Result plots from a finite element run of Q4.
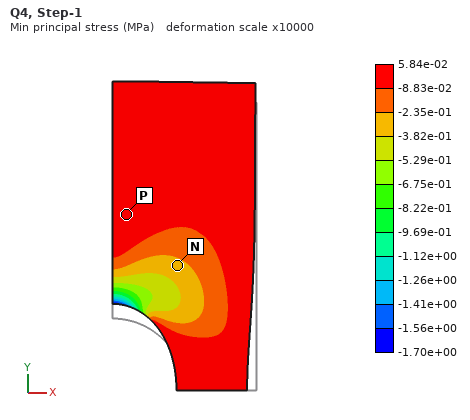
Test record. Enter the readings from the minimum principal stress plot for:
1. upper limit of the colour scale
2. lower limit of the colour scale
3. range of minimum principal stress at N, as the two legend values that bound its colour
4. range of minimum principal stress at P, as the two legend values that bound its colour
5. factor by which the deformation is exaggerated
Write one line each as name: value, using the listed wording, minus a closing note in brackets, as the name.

upper limit of the colour scale: 5.84e-02 MPa
lower limit of the colour scale: -1.70e+00 MPa
range of minimum principal stress at N, as the two legend values that bound its colour: -3.82e-01 to -2.35e-01 MPa
range of minimum principal stress at P, as the two legend values that bound its colour: -8.83e-02 to 5.84e-02 MPa
factor by which the deformation is exaggerated: 10000
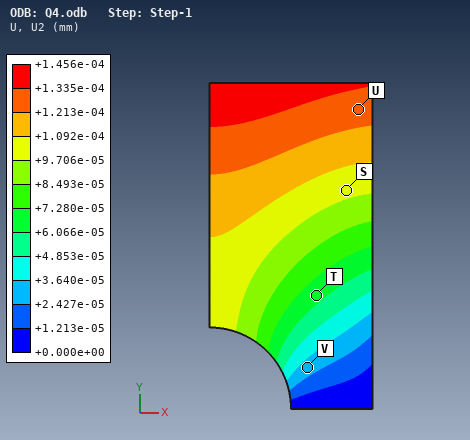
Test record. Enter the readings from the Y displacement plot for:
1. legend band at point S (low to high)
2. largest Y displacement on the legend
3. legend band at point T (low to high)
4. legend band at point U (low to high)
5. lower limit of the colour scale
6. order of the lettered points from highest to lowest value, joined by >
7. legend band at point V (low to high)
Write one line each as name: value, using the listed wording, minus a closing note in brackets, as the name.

legend band at point S: +9.706e-05 to +1.092e-04 mm
largest Y displacement on the legend: +1.456e-04 mm
legend band at point T: +6.066e-05 to +7.280e-05 mm
legend band at point U: +1.213e-04 to +1.335e-04 mm
lower limit of the colour scale: +0.000e+00 mm
order of the lettered points from highest to lowest value, joined by >: U > S > T > V
legend band at point V: +2.427e-05 to +3.640e-05 mm
